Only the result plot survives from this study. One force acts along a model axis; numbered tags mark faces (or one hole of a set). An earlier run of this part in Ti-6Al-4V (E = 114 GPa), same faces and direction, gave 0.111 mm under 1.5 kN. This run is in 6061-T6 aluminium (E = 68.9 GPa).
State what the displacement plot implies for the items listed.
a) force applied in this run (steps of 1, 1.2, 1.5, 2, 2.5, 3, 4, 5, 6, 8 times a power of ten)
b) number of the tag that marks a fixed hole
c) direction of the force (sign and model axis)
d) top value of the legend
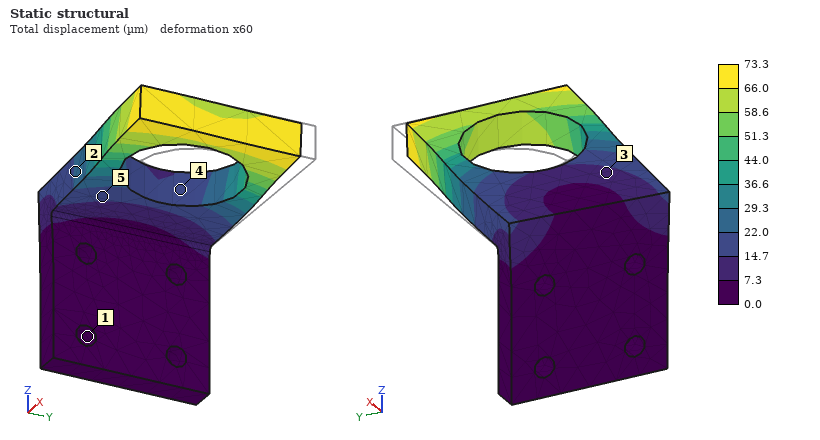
600 N
1
-Y
73.3 µm
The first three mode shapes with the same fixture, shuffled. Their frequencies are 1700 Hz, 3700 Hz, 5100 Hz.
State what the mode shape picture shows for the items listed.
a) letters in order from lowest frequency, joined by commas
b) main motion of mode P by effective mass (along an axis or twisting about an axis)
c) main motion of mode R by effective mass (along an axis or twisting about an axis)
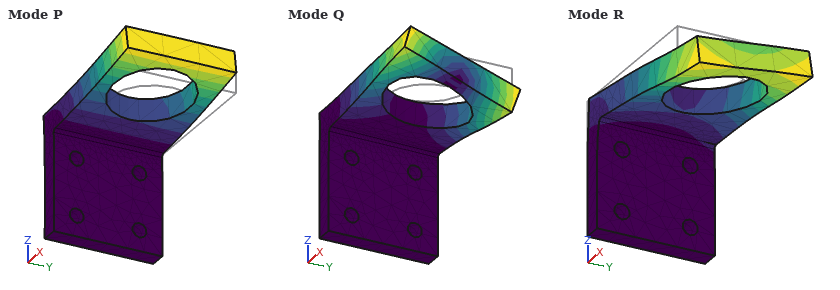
P, R, Q
along Z
along Y
